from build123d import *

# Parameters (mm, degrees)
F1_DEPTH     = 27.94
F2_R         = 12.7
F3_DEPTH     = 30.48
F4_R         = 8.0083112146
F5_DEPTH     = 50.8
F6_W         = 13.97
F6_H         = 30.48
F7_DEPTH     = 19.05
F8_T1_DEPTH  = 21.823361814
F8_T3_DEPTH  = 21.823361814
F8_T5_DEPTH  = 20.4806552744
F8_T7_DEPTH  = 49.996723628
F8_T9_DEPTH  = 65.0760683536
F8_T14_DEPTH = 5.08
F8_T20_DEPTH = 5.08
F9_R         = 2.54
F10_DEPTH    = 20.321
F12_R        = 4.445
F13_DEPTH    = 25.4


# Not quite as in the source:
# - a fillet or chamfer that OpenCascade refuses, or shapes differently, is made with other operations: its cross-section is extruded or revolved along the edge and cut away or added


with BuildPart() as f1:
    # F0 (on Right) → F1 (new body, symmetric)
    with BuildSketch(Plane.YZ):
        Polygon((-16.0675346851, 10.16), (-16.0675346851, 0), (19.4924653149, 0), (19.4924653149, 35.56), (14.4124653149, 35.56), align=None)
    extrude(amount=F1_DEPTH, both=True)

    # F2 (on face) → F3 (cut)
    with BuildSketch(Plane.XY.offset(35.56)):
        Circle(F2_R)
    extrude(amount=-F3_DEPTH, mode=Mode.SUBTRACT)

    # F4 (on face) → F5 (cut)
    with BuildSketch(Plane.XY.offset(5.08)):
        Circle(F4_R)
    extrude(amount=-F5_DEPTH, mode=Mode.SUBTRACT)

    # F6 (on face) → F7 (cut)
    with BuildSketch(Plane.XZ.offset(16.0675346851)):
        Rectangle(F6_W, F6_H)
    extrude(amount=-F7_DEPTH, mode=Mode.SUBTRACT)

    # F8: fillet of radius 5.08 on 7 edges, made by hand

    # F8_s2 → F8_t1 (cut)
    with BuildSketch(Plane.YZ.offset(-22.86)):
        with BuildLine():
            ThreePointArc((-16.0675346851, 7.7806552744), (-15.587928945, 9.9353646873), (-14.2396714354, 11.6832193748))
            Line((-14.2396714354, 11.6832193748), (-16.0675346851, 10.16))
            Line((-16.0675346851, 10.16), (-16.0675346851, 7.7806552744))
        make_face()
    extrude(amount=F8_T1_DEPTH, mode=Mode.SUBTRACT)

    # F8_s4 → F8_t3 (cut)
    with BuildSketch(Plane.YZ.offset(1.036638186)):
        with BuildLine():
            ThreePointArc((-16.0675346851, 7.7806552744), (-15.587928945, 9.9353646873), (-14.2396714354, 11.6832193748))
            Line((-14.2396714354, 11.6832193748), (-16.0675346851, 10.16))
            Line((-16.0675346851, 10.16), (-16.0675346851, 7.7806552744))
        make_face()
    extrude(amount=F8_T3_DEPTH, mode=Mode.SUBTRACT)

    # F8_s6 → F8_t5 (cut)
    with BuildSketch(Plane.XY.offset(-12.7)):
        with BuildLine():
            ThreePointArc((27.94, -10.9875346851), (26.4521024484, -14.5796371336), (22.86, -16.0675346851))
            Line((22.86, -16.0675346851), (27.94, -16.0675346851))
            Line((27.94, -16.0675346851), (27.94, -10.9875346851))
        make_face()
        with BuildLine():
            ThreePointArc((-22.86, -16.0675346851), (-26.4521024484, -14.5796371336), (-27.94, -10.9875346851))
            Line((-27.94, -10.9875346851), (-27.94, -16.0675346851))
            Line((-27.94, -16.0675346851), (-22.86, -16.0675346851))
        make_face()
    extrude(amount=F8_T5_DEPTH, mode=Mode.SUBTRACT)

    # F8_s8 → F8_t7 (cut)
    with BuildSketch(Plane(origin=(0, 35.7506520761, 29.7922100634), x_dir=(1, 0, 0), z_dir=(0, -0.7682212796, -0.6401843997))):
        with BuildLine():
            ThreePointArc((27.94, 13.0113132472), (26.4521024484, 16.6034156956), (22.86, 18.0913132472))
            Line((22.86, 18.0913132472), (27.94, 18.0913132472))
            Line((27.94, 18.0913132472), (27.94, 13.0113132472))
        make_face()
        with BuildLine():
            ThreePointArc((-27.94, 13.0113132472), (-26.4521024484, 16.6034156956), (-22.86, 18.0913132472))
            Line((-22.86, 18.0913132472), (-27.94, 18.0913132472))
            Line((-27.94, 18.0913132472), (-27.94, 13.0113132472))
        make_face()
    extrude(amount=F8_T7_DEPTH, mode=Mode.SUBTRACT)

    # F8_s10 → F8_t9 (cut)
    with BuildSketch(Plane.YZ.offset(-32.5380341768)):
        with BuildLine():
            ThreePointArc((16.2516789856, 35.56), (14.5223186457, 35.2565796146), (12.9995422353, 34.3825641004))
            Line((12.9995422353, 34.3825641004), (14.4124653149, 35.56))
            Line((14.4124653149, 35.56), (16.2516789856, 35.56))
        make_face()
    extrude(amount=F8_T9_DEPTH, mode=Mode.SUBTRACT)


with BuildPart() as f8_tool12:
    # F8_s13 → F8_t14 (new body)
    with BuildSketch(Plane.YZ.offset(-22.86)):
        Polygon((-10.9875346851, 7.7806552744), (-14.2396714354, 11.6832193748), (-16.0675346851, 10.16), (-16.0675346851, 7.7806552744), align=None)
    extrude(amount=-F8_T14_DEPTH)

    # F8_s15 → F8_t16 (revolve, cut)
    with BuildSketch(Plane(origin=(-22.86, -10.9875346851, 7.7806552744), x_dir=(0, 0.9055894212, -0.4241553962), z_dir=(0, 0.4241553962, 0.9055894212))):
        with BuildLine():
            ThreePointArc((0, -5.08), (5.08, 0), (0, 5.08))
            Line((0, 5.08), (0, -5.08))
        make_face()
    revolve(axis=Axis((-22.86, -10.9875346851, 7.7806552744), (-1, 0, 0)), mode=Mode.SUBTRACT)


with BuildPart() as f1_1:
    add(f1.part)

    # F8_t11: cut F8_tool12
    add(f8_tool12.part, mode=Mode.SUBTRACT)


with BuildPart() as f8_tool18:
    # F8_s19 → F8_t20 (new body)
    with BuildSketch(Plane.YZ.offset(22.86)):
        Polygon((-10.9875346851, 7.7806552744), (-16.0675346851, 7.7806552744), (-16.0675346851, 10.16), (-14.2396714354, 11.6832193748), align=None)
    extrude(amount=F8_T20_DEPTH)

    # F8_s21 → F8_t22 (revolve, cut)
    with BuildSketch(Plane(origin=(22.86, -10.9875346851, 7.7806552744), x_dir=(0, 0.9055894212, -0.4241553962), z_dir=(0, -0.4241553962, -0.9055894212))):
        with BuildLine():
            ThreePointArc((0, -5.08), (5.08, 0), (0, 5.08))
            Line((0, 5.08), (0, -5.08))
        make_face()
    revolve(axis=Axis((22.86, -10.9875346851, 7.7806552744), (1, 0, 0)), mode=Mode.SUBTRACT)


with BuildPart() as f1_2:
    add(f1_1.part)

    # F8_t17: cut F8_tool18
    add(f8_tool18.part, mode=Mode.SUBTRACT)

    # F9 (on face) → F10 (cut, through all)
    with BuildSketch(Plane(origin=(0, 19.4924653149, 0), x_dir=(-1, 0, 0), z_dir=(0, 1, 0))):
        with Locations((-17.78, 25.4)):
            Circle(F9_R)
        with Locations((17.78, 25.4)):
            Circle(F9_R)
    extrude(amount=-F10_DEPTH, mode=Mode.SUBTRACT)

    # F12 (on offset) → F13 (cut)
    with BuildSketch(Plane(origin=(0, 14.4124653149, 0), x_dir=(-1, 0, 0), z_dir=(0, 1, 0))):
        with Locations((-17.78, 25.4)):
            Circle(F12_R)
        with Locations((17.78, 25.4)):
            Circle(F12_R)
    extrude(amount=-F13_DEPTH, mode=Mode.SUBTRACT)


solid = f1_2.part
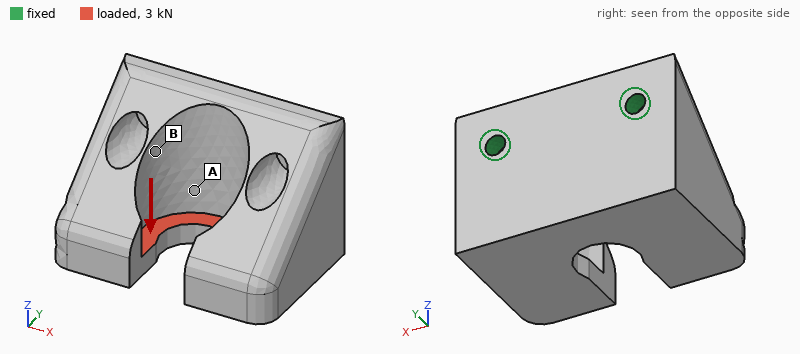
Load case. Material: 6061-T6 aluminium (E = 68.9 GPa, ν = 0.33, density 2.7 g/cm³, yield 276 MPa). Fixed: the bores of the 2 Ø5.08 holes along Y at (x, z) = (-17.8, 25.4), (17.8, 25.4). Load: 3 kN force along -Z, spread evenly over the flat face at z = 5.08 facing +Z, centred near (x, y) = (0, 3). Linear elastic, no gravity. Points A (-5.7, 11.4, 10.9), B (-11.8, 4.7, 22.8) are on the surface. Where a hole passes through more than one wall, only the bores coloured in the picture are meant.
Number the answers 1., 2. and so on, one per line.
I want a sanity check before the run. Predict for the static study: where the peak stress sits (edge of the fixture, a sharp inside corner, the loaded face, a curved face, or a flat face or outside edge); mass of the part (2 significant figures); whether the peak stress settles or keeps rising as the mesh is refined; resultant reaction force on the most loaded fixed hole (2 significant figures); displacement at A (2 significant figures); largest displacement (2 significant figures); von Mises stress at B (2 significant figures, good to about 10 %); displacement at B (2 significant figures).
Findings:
1. edge of the fixture
2. 95 g
3. keeps rising
4. 1.5 kN
5. 0.044 mm
6. 0.13 mm
7. 38 MPa
8. 0.036 mm
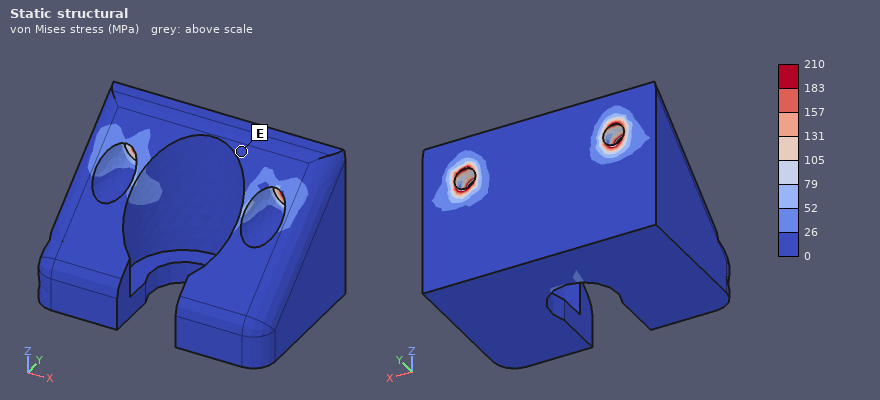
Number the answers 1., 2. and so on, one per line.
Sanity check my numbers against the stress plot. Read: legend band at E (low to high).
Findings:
1. 0 to 26 MPa
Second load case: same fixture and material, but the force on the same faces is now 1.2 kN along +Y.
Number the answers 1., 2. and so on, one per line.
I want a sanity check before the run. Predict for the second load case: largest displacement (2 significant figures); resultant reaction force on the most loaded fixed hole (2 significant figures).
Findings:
1. 71 µm
2. 620 N
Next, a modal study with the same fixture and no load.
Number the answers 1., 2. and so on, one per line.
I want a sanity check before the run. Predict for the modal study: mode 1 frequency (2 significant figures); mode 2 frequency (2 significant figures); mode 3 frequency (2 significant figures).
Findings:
1. 3000 Hz
2. 5300 Hz
3. 6800 Hz
